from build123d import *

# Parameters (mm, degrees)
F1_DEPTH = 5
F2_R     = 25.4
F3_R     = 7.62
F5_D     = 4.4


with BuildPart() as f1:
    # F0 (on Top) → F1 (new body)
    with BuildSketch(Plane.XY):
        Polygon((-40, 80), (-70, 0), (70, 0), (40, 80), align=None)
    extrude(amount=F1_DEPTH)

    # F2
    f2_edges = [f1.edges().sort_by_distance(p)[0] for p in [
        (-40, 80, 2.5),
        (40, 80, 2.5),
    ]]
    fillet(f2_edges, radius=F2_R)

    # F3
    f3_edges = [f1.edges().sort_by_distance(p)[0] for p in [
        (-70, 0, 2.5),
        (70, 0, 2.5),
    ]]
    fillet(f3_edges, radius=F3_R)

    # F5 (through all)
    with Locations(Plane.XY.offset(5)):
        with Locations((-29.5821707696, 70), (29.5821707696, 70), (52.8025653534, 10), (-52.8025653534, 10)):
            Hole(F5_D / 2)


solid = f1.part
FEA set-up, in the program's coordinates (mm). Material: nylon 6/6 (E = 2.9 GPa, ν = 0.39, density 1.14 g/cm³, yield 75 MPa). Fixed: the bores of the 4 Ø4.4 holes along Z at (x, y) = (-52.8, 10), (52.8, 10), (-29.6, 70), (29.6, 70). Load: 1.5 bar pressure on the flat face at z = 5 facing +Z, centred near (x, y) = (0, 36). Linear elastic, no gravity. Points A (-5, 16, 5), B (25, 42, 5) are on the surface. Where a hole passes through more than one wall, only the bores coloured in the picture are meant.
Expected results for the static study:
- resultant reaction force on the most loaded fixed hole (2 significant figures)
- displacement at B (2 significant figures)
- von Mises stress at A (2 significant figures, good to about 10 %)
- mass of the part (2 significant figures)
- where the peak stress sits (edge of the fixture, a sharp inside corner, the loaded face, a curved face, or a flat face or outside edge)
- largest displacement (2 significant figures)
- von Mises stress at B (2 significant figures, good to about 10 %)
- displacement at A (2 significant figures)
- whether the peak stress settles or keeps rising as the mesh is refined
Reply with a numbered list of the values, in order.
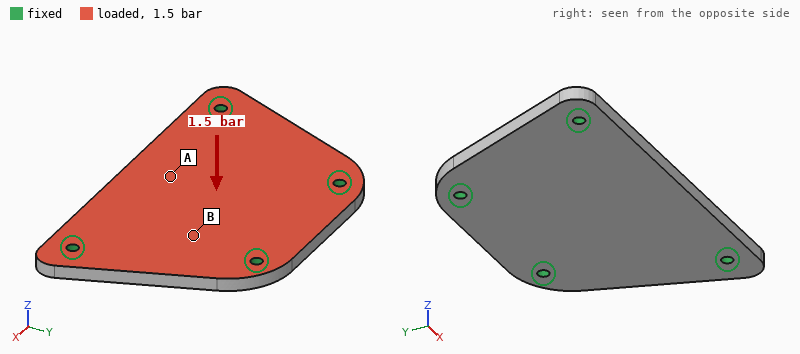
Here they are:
1. 340 N
2. 0.66 mm
3. 13 MPa
4. 49 g
5. edge of the fixture
6. 1.8 mm
7. 7.0 MPa
8. 1.5 mm
9. keeps rising
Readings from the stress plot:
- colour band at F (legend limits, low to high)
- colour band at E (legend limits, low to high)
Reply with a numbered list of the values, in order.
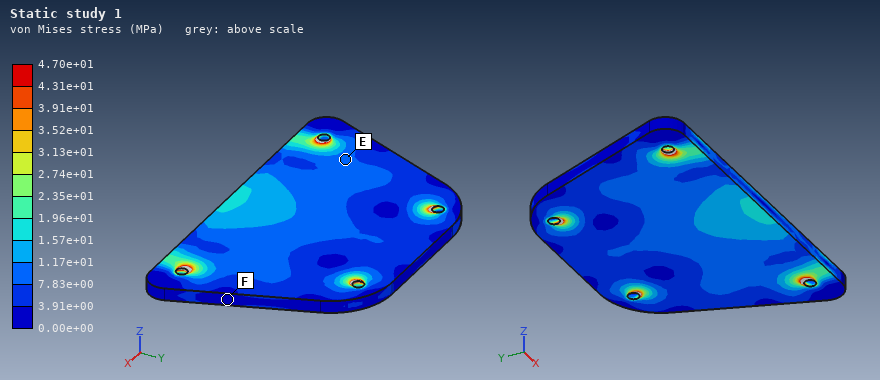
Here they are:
1. 0.00e+00 to 3.91e+00 MPa
2. 7.83e+00 to 1.17e+01 MPa
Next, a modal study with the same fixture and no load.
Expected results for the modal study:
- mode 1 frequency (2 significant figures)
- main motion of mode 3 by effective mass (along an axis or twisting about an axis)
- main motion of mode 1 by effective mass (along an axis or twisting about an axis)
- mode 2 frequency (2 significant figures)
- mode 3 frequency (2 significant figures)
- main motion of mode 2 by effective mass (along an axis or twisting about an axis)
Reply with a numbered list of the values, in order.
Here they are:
1. 790 Hz
2. twisting about Y
3. along Z
4. 1700 Hz
5. 1800 Hz
6. along Z
